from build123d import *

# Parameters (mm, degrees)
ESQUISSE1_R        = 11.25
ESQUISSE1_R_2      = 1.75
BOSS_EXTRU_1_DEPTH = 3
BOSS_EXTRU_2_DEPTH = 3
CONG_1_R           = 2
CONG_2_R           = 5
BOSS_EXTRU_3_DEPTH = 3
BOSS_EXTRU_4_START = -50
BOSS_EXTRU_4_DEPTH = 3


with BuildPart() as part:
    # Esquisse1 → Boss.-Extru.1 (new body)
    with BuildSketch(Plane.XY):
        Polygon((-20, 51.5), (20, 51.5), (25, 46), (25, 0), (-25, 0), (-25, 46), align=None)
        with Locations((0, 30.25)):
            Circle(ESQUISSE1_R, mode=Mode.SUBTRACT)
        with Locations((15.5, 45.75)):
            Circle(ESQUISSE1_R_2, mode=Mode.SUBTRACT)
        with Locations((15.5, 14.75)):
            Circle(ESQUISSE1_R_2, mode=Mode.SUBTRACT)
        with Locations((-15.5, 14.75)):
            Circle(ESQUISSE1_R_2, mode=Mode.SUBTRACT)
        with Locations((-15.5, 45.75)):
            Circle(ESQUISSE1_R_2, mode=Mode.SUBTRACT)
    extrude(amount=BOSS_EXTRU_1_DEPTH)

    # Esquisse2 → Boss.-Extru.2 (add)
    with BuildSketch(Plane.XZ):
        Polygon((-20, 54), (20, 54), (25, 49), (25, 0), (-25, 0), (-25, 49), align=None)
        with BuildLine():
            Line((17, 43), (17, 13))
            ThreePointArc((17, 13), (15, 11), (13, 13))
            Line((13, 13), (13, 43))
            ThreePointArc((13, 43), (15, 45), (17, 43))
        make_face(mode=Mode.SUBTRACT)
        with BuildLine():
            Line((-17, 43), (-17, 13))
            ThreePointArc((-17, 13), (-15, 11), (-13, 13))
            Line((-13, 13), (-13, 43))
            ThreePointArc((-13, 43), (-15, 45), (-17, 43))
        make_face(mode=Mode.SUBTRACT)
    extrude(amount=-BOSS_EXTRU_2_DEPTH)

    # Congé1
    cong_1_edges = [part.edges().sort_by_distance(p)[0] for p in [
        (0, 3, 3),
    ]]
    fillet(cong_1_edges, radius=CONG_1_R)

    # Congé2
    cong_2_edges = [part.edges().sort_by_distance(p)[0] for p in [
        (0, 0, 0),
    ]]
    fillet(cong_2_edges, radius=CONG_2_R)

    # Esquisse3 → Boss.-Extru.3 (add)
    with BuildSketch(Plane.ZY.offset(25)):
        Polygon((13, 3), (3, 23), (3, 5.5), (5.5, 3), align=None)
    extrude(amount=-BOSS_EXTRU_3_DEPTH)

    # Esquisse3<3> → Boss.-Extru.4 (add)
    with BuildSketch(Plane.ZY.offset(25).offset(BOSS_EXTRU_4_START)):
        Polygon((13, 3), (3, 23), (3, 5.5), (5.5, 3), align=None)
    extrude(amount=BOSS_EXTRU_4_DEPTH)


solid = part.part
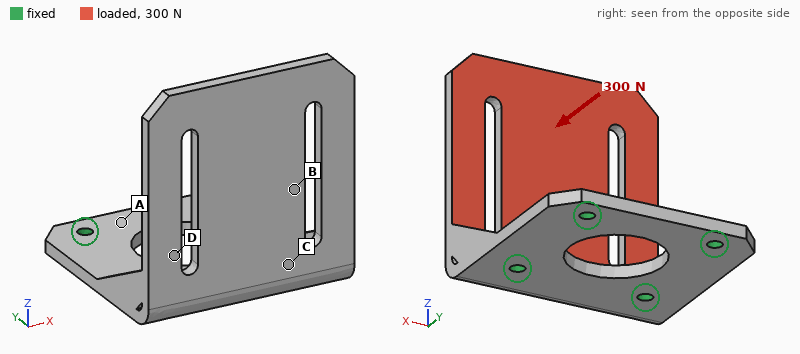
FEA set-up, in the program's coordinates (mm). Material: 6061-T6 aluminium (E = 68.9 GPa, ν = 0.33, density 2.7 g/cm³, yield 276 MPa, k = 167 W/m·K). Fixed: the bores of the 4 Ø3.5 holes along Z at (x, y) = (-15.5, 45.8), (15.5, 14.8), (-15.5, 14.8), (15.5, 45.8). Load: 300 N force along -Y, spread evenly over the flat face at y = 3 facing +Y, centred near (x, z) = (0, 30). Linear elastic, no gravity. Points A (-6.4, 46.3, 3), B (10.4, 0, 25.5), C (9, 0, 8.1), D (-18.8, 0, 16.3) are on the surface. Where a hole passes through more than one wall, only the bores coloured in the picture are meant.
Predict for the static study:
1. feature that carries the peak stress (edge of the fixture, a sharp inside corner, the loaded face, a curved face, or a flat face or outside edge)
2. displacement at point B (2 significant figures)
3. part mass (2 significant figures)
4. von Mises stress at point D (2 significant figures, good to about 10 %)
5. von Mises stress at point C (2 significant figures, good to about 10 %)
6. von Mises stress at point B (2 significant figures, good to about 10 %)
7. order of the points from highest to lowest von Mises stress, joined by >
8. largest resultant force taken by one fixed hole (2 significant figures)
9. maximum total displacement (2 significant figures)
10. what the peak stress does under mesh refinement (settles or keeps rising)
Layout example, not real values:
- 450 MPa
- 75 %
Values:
- edge of the fixture
- 0.32 mm
- 36 g
- 95 MPa
- 63 MPa
- 31 MPa
- D > C > B > A
- 170 N
- 0.93 mm
- keeps rising
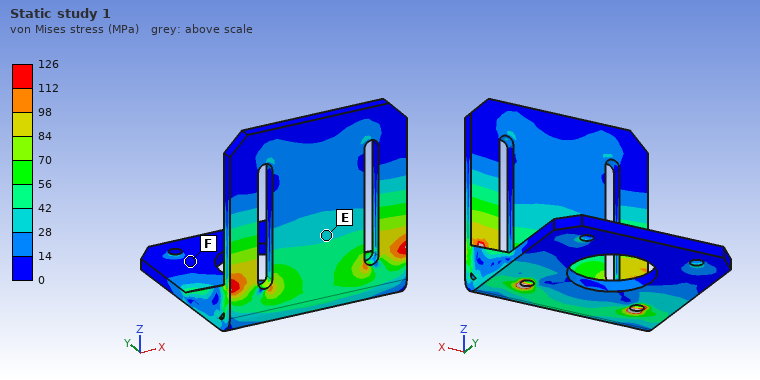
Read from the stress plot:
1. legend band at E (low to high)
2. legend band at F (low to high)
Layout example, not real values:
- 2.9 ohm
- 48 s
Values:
- 28 to 42 MPa
- 0 to 14 MPa
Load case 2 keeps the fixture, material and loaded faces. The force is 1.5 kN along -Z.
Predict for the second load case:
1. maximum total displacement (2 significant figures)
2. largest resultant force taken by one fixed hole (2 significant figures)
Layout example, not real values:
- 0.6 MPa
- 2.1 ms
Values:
- 0.23 mm
- 840 N
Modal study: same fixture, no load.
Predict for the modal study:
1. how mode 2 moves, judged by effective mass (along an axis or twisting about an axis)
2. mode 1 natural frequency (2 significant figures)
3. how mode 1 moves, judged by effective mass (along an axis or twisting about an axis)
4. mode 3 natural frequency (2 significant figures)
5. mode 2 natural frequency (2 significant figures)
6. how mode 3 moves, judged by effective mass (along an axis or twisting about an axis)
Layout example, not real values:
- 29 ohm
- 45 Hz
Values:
- along X
- 860 Hz
- along Y
- 3000 Hz
- 2000 Hz
- along X
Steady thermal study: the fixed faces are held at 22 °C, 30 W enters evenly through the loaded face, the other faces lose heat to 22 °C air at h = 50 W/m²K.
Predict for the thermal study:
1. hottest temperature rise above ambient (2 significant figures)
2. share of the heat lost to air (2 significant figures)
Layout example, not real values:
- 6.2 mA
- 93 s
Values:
- 42 K
- 20 %
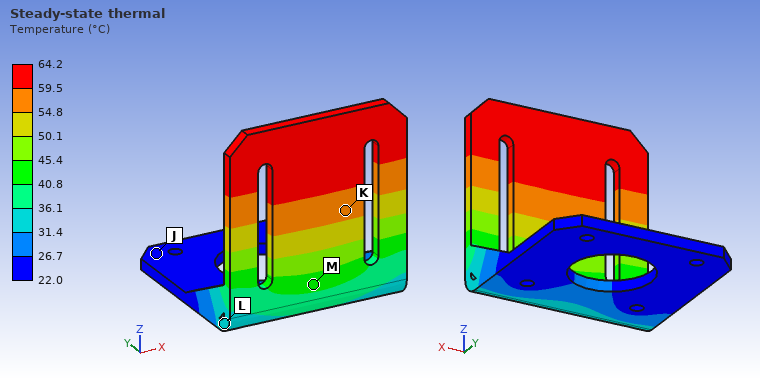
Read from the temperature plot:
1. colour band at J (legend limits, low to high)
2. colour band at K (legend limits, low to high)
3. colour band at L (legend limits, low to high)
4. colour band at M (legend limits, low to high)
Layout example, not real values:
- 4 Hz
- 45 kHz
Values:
- 22.0 to 26.7 °C
- 54.8 to 59.5 °C
- 31.4 to 36.1 °C
- 40.8 to 45.4 °C
